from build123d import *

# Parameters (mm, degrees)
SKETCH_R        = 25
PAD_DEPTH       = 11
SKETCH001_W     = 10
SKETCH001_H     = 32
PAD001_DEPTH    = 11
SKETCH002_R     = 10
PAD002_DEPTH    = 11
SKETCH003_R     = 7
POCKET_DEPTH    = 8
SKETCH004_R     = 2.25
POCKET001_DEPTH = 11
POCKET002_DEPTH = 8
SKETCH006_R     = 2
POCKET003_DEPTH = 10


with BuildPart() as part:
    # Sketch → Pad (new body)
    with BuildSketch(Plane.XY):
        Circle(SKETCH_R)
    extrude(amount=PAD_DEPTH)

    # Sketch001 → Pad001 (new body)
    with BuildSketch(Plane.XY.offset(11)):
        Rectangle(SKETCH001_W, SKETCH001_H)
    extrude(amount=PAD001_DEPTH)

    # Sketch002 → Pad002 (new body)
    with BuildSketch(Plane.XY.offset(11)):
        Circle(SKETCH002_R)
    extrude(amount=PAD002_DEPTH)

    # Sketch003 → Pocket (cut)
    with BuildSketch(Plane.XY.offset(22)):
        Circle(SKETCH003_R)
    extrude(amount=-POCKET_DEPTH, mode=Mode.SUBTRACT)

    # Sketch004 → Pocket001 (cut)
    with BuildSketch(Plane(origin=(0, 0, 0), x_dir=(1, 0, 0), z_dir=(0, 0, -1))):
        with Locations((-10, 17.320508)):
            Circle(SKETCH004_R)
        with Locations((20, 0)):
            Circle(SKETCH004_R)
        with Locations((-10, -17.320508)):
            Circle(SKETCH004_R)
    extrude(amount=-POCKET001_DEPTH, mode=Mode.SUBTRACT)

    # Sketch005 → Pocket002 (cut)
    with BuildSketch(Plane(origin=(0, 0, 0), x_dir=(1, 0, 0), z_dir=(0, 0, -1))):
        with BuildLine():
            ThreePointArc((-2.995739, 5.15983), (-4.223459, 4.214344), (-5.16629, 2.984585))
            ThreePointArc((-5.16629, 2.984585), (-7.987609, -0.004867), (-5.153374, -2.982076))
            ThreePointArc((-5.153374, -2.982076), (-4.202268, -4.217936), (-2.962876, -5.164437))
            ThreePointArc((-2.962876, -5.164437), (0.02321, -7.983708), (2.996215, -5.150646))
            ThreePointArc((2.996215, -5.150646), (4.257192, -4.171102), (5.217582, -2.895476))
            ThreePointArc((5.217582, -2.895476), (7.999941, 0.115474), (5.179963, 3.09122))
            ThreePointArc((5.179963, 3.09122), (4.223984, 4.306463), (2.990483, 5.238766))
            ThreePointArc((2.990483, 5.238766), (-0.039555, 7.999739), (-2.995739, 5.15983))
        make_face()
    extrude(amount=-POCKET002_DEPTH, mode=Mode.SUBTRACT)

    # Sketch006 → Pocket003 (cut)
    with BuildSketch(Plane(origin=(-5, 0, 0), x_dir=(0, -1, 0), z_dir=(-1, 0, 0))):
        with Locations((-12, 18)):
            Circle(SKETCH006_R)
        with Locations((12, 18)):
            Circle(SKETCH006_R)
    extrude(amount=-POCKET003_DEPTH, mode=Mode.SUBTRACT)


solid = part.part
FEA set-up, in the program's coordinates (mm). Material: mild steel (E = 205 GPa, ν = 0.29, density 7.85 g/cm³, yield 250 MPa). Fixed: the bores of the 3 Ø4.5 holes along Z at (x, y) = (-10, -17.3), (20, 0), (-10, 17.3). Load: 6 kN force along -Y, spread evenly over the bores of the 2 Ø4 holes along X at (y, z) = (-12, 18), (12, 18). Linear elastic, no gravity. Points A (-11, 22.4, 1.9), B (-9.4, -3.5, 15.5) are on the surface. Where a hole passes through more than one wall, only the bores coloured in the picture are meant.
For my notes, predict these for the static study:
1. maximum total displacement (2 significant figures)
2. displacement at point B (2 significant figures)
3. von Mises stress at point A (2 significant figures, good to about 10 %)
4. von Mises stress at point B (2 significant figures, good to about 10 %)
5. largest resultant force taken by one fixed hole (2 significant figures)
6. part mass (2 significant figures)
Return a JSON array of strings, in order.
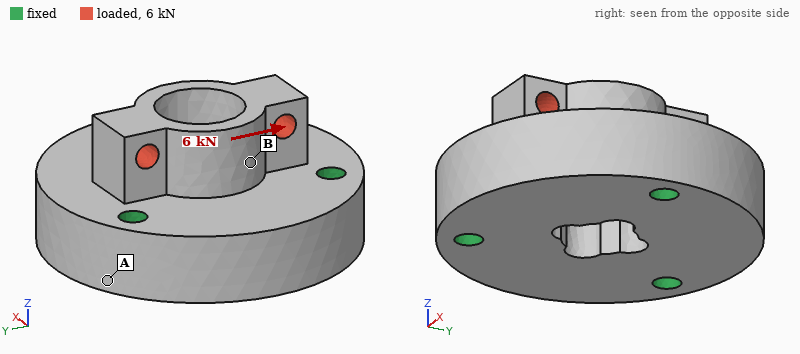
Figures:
["8.4 µm", "3.4 µm", "13 MPa", "37 MPa", "2.9 kN", "180 g"]
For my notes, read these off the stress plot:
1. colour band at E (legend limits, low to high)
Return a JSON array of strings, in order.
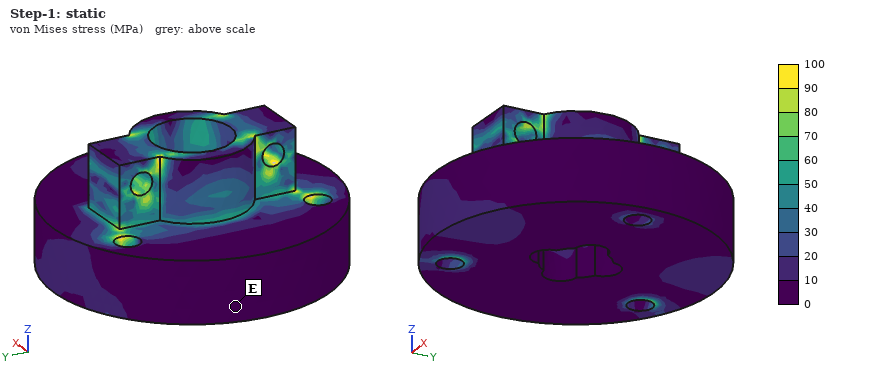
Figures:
["0 to 10 MPa"]
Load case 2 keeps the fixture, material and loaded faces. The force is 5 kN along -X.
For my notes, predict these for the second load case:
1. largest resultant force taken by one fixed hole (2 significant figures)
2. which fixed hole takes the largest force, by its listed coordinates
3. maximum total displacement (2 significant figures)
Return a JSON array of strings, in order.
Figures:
["2.5 kN", "(20, 0)", "9.0 µm"]
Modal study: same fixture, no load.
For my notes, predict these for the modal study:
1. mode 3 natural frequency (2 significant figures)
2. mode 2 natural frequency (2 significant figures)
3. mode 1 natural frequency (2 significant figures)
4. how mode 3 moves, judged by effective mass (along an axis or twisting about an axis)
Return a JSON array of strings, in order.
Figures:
["24 kHz", "23 kHz", "22 kHz", "along Z"]
